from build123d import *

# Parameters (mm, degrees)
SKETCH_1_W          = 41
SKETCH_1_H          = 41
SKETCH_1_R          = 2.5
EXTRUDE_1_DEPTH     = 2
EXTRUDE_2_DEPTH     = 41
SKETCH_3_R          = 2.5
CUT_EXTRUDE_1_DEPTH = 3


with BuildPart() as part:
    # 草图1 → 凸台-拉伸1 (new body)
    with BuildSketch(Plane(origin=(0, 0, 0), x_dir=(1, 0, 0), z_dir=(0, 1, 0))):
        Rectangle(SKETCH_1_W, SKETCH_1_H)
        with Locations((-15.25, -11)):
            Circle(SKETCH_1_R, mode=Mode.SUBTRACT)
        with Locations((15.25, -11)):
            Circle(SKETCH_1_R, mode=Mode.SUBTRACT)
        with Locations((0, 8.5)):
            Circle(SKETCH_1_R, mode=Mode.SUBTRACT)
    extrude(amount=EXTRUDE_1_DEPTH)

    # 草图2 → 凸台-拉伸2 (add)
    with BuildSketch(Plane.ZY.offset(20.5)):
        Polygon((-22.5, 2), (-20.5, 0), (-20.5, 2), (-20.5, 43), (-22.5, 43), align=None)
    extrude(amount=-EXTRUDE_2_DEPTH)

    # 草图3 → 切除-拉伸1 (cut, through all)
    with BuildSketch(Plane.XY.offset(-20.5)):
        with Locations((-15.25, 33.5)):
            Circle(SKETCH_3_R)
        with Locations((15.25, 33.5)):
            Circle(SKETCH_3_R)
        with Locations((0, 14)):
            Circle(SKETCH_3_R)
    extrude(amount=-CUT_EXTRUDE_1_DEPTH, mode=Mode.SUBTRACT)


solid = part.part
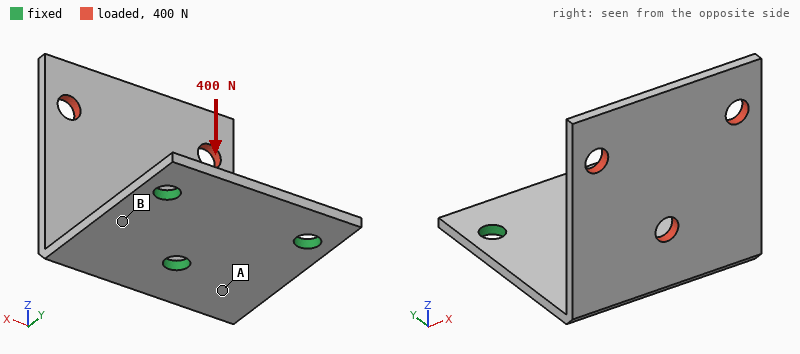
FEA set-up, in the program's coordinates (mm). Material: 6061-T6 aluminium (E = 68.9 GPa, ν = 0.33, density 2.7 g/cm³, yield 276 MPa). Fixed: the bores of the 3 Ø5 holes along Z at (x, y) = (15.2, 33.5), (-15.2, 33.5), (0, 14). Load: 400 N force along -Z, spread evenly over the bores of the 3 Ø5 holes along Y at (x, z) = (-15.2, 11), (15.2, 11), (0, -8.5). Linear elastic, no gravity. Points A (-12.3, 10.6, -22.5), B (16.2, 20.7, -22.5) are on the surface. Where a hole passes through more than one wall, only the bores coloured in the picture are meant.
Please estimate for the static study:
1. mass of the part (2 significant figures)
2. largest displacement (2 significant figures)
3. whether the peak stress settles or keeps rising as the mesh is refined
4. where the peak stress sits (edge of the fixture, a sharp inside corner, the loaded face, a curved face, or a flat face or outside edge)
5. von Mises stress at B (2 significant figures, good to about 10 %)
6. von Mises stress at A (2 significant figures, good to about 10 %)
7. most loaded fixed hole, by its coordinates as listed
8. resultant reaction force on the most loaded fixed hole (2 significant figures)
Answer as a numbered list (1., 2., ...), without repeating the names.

1. 18 g
2. 0.78 mm
3. keeps rising
4. edge of the fixture
5. 32 MPa
6. 75 MPa
7. (0, 14)
8. 480 N
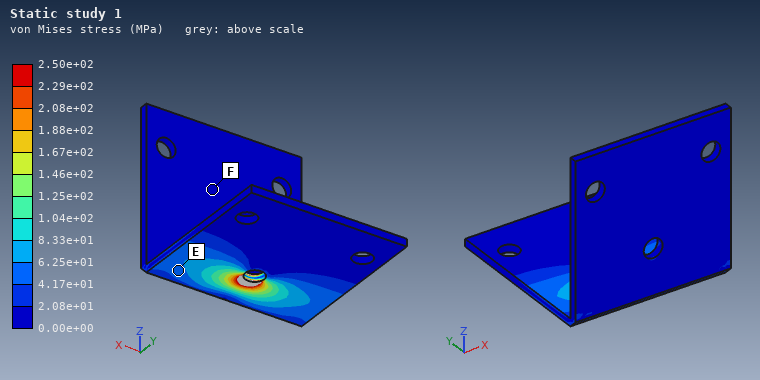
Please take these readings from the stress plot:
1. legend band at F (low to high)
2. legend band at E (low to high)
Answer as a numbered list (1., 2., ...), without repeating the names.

1. 0.00e+00 to 2.08e+01 MPa
2. 4.17e+01 to 6.25e+01 MPa
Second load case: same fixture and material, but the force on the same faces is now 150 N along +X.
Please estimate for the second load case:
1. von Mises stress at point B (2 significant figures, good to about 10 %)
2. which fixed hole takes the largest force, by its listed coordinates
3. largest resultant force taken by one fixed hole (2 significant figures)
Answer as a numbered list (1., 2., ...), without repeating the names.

1. 57 MPa
2. (0, 14)
3. 160 N
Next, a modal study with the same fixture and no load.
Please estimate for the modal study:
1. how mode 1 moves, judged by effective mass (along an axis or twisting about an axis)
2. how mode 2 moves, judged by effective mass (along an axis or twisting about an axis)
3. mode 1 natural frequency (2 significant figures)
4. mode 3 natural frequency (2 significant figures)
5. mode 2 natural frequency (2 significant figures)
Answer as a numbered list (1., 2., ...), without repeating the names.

1. along Y
2. along X
3. 630 Hz
4. 2100 Hz
5. 1000 Hz
